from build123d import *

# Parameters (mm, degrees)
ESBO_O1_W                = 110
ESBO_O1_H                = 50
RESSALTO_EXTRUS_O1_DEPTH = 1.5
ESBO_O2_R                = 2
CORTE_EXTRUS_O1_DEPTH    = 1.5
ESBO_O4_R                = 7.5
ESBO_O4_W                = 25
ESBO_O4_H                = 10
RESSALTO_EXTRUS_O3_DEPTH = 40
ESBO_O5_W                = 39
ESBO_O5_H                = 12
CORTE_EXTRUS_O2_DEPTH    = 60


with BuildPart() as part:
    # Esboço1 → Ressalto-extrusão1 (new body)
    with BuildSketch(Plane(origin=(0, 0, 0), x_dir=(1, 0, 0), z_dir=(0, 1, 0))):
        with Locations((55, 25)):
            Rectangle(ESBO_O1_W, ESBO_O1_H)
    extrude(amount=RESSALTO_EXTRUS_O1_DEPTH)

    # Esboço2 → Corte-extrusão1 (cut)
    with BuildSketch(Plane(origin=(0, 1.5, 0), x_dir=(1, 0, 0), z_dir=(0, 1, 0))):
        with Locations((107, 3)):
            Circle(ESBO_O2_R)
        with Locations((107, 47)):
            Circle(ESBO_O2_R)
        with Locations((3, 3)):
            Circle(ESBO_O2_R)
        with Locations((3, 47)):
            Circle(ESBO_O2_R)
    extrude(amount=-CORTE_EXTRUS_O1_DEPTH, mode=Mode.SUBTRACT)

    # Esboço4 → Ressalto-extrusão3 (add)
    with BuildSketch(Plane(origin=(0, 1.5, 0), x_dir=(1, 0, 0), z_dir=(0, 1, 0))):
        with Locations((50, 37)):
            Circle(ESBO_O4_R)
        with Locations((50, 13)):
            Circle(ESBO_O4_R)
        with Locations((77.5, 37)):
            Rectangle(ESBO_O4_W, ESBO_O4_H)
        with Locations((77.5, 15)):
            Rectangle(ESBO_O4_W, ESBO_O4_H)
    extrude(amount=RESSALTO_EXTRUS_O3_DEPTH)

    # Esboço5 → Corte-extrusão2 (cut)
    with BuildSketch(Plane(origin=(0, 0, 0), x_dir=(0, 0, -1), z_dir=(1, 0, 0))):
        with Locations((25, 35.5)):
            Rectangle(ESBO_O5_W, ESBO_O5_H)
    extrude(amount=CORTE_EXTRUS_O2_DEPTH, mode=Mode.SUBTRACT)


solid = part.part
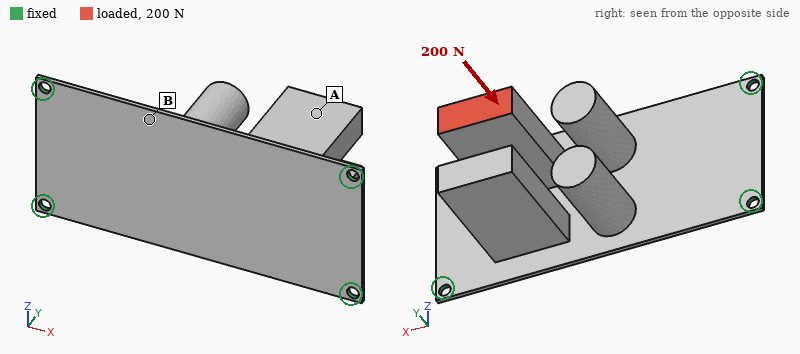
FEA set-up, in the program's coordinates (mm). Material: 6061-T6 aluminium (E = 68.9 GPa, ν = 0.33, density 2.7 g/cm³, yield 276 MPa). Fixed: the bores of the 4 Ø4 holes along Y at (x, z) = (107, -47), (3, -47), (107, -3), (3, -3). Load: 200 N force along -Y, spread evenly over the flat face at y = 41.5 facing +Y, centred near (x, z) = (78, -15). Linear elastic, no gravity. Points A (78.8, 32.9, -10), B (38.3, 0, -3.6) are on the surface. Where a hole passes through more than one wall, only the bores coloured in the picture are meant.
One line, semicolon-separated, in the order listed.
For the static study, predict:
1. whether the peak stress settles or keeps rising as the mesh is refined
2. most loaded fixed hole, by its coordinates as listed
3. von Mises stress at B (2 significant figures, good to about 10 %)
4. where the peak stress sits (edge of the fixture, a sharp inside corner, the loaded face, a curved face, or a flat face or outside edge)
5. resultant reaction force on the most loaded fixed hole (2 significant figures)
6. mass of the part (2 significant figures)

keeps rising; (107, -3); 39 MPa; edge of the fixture; 130 N; 100 g
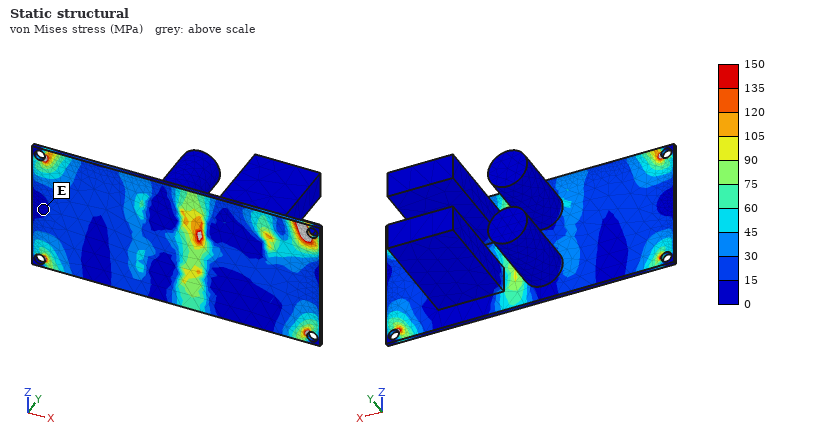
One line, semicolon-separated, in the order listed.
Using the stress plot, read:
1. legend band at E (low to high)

0 to 15 MPa
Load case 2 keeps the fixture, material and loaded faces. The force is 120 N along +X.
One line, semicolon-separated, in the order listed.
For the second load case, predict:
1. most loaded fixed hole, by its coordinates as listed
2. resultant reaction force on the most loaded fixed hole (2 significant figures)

(3, -47); 56 N
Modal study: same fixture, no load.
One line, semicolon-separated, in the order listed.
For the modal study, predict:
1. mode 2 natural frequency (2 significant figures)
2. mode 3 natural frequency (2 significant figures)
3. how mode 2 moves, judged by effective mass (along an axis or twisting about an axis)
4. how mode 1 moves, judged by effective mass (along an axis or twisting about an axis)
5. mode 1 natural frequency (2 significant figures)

430 Hz; 560 Hz; along Z; along Y; 270 Hz
